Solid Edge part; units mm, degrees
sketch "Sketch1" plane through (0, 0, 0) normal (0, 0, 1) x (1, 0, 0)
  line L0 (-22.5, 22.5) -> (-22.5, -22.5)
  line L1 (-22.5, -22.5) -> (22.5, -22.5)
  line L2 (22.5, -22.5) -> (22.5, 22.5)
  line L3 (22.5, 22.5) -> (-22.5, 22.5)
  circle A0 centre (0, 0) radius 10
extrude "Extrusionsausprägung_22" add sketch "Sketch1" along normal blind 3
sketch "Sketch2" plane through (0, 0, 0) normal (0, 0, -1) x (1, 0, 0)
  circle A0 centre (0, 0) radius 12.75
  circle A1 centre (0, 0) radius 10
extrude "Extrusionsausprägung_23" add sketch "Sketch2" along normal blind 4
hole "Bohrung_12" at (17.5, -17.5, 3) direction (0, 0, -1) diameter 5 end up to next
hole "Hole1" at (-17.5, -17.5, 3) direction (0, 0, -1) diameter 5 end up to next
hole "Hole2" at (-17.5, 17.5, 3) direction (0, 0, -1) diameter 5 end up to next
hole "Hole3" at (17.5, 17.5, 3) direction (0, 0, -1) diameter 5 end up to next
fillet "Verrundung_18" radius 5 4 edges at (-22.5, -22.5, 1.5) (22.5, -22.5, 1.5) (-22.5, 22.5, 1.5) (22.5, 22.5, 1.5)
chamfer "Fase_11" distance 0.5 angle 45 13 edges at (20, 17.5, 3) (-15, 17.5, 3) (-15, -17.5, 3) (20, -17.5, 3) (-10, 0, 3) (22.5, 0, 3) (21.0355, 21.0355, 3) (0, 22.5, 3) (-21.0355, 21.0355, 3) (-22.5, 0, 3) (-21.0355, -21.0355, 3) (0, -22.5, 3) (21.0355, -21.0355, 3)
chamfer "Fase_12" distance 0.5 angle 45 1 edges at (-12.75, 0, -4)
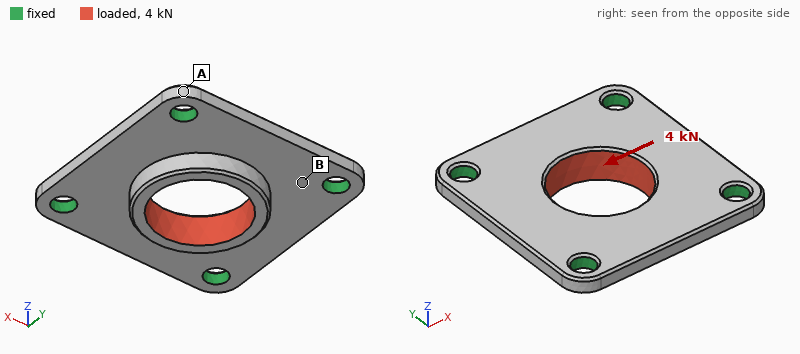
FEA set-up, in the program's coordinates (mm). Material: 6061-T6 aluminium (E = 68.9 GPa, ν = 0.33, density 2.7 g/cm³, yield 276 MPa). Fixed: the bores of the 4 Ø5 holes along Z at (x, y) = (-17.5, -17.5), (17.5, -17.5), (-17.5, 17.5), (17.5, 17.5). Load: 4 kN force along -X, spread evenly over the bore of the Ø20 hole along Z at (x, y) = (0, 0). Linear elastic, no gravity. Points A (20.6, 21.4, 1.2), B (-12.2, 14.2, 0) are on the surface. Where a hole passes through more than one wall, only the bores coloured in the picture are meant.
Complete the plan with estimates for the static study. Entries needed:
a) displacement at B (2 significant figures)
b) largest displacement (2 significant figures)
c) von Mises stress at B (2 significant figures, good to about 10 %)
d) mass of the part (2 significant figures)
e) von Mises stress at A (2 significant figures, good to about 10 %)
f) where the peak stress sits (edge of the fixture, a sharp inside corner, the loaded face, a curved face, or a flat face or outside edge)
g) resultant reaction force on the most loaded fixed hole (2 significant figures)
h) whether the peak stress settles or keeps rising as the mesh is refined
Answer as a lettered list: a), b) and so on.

a) 3.5 µm
b) 21 µm
c) 39 MPa
d) 15 g
e) 8.4 MPa
f) edge of the fixture
g) 1.1 kN
h) keeps rising
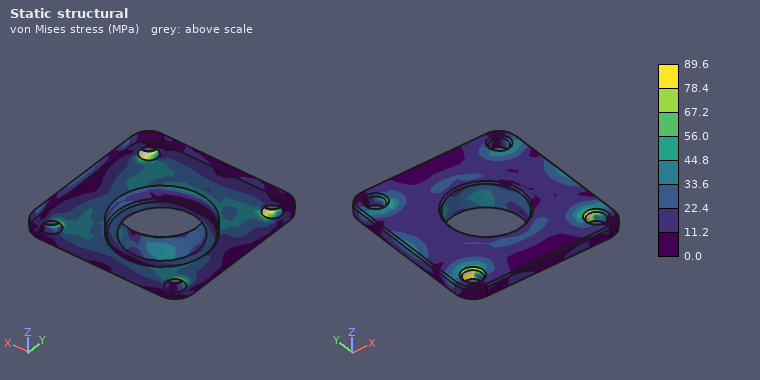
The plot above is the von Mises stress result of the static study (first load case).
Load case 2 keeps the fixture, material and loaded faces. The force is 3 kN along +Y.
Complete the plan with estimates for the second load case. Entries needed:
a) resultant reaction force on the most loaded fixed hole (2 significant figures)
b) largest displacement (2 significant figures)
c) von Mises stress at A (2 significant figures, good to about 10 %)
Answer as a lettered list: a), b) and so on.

a) 810 N
b) 15 µm
c) 6.8 MPa
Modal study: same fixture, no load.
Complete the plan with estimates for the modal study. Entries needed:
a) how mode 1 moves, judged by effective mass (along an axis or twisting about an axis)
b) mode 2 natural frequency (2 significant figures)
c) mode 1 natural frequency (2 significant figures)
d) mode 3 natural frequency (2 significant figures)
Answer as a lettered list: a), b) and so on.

a) along Z
b) 15 kHz
c) 12 kHz
d) 15 kHz
